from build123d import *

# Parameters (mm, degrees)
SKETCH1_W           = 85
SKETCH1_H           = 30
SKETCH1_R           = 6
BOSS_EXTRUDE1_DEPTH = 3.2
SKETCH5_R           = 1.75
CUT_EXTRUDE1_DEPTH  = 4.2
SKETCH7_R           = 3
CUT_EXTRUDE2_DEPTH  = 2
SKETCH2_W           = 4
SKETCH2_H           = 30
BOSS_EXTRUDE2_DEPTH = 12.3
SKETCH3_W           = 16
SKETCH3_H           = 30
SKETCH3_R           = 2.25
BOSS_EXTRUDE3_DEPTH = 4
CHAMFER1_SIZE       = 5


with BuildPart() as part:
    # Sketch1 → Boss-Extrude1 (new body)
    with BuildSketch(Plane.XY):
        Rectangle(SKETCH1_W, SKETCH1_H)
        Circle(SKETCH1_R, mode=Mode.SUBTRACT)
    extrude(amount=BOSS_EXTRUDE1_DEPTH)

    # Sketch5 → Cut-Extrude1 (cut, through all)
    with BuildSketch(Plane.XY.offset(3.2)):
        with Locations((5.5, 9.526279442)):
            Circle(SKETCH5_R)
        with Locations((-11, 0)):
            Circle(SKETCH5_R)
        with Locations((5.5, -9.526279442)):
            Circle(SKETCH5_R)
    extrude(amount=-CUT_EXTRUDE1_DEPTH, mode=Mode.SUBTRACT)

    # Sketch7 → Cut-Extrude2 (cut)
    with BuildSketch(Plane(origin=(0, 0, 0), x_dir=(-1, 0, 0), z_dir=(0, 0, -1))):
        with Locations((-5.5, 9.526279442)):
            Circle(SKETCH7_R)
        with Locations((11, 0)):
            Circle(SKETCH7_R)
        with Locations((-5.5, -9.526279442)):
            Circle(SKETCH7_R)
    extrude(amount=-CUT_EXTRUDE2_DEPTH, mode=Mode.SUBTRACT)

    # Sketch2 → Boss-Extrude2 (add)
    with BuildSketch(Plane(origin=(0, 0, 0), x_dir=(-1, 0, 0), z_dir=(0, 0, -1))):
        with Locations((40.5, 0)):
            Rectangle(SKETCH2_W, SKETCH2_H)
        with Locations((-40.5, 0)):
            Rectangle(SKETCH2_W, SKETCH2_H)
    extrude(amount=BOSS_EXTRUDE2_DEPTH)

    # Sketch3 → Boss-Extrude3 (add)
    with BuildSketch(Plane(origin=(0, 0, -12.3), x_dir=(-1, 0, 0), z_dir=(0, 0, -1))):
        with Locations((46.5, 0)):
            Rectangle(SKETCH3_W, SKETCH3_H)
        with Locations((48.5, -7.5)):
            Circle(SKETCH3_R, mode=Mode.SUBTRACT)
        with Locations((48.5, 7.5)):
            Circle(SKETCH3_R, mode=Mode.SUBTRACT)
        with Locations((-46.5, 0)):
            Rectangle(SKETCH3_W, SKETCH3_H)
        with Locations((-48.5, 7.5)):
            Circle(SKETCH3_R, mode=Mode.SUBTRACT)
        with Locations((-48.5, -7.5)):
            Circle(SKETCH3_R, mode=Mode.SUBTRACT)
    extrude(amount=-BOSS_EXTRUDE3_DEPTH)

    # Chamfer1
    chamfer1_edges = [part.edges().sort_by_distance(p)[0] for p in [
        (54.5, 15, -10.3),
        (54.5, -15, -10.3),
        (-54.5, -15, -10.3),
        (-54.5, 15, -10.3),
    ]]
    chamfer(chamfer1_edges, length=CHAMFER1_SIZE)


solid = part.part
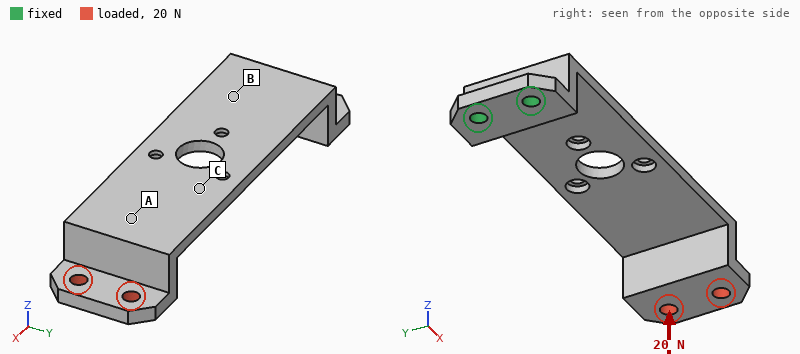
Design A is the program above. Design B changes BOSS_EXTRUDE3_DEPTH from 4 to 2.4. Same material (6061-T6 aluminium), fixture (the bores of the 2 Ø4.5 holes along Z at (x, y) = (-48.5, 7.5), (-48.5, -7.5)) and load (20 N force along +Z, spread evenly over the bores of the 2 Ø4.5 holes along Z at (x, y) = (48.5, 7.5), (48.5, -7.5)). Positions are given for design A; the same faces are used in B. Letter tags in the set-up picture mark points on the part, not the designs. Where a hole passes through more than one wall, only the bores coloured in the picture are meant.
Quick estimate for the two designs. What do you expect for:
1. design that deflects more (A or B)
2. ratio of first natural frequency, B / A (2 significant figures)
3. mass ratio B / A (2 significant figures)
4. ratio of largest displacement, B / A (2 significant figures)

B
0.92
0.93
1.3
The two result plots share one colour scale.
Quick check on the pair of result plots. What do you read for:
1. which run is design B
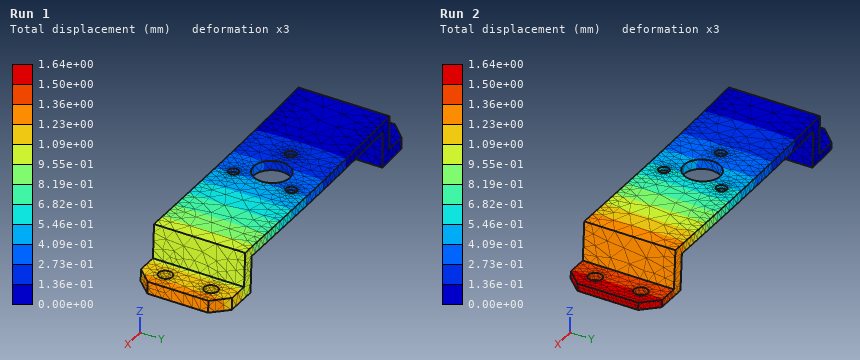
Run 2
